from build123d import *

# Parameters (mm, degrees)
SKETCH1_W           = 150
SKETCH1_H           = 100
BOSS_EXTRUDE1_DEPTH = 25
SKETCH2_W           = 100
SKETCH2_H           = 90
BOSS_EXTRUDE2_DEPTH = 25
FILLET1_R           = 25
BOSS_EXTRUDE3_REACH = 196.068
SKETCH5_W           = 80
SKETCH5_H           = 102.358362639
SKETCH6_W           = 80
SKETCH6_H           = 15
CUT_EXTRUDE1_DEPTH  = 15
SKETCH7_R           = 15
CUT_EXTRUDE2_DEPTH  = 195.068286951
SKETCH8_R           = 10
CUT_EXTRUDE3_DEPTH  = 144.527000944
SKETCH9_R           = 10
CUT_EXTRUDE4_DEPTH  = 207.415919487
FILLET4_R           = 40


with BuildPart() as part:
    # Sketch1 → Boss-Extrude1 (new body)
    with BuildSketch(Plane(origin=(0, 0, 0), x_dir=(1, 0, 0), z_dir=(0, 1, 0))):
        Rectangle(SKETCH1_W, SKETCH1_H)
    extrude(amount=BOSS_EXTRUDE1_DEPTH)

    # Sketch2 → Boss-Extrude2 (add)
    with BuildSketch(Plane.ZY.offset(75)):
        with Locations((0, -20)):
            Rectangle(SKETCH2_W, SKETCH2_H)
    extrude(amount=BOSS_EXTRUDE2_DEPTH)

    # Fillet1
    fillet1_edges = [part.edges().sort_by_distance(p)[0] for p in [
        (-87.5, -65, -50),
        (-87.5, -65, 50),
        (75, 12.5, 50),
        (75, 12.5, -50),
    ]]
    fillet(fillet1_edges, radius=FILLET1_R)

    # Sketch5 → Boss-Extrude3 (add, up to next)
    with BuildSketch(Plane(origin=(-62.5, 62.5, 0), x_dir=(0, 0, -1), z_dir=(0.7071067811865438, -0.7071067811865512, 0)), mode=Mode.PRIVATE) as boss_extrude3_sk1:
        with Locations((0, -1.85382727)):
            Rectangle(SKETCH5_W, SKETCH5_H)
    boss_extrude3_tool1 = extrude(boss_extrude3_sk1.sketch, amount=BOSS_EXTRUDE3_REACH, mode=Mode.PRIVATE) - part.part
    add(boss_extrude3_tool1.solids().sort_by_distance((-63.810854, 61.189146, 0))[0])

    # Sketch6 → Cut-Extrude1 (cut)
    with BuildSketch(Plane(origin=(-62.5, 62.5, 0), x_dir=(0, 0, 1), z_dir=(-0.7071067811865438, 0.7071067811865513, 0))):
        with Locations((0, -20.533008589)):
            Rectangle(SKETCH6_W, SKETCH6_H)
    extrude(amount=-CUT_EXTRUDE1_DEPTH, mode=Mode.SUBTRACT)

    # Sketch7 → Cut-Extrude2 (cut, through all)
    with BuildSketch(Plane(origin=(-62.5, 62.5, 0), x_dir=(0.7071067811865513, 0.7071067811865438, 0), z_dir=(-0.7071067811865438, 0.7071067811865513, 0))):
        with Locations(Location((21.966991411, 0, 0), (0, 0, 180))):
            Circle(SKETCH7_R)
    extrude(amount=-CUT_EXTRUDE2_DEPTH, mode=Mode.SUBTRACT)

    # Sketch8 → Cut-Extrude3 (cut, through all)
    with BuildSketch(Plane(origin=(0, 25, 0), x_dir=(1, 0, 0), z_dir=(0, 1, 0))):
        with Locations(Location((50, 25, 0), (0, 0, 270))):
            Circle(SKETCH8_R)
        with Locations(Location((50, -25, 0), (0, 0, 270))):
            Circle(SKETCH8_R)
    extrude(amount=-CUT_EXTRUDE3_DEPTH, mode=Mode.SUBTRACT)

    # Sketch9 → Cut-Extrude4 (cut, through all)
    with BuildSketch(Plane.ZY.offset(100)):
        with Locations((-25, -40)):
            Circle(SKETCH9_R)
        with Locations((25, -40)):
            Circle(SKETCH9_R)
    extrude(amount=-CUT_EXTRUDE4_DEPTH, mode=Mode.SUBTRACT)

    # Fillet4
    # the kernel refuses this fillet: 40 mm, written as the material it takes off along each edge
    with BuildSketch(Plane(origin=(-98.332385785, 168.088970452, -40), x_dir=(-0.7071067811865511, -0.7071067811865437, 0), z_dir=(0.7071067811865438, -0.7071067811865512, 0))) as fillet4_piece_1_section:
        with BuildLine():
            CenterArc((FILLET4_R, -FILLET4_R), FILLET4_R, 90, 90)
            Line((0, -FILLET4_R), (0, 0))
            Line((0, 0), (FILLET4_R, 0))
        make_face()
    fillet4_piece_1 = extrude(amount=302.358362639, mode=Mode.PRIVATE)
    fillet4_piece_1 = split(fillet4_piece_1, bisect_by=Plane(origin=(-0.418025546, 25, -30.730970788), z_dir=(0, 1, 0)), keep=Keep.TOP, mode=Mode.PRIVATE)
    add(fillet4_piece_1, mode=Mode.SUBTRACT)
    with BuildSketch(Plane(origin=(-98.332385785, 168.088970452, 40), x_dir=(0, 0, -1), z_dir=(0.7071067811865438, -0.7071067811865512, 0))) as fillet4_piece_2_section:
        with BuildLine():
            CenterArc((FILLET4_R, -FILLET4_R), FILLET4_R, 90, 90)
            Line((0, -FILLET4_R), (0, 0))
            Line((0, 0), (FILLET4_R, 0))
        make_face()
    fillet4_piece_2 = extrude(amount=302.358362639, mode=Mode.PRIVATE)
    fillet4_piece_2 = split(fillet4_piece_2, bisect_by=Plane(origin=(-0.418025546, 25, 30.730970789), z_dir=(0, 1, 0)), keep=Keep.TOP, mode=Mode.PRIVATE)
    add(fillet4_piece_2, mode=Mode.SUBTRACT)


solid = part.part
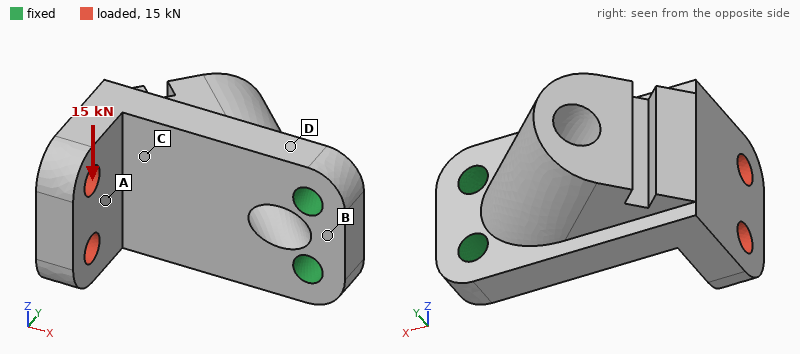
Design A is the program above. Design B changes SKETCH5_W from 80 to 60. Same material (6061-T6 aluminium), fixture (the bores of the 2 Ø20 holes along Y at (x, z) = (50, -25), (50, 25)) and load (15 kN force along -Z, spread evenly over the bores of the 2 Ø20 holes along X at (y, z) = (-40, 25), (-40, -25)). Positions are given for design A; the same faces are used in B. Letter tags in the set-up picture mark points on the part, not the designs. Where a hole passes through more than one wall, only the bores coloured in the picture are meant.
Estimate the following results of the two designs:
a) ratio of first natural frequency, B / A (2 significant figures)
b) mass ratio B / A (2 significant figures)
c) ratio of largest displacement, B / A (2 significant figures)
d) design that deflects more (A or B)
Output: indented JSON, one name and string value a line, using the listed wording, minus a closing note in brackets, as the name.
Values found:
{
  "ratio of first natural frequency, B / A": "1.0",
  "mass ratio B / A": "0.93",
  "ratio of largest displacement, B / A": "1.1",
  "design that deflects more": "B"
}
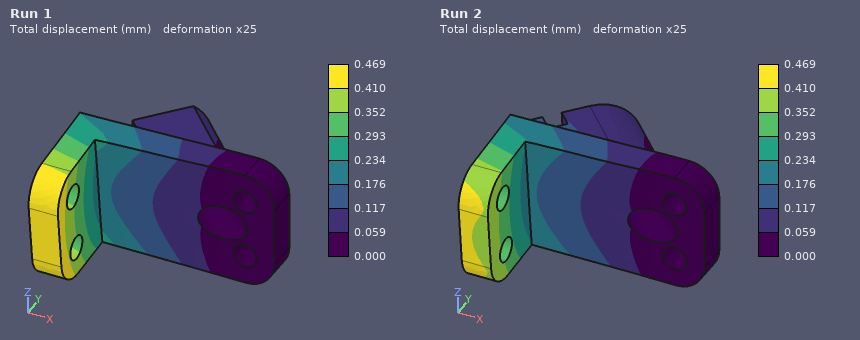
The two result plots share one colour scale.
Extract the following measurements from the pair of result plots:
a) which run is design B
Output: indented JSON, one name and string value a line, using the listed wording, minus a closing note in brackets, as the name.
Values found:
{
  "which run is design B": "Run 1"
}
